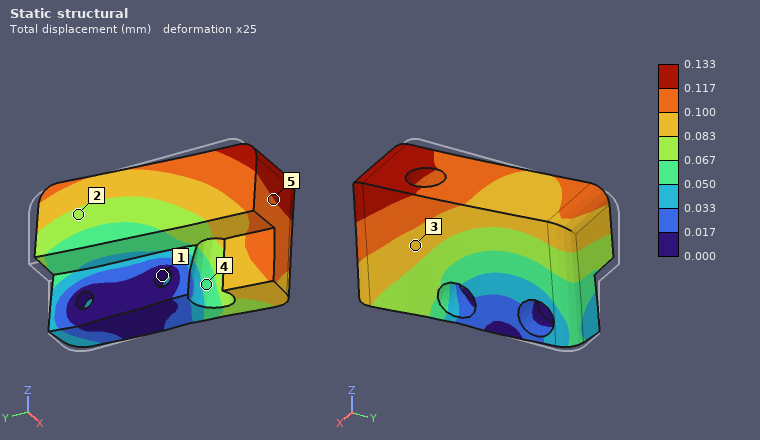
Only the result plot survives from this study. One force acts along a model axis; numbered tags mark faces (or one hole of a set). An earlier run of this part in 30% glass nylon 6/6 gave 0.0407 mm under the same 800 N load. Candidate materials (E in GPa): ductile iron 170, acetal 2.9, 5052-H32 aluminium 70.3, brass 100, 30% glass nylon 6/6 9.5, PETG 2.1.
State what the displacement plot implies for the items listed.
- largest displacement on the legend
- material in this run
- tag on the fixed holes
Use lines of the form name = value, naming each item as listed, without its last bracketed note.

largest displacement on the legend = 0.133 mm
material in this run = acetal
tag on the fixed holes = 1
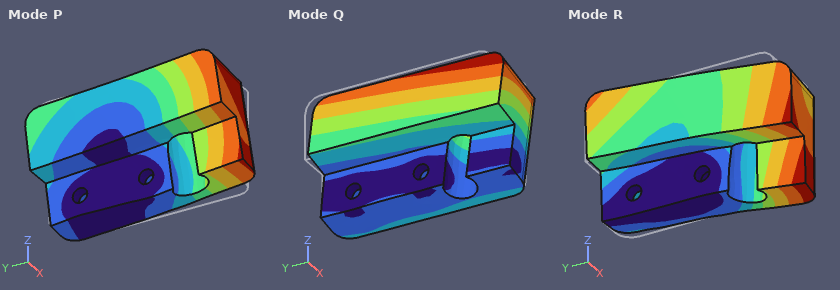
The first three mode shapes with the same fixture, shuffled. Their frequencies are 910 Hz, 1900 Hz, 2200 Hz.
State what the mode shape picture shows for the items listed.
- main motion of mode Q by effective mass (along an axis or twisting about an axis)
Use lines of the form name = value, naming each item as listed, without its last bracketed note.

main motion of mode Q by effective mass = along X
